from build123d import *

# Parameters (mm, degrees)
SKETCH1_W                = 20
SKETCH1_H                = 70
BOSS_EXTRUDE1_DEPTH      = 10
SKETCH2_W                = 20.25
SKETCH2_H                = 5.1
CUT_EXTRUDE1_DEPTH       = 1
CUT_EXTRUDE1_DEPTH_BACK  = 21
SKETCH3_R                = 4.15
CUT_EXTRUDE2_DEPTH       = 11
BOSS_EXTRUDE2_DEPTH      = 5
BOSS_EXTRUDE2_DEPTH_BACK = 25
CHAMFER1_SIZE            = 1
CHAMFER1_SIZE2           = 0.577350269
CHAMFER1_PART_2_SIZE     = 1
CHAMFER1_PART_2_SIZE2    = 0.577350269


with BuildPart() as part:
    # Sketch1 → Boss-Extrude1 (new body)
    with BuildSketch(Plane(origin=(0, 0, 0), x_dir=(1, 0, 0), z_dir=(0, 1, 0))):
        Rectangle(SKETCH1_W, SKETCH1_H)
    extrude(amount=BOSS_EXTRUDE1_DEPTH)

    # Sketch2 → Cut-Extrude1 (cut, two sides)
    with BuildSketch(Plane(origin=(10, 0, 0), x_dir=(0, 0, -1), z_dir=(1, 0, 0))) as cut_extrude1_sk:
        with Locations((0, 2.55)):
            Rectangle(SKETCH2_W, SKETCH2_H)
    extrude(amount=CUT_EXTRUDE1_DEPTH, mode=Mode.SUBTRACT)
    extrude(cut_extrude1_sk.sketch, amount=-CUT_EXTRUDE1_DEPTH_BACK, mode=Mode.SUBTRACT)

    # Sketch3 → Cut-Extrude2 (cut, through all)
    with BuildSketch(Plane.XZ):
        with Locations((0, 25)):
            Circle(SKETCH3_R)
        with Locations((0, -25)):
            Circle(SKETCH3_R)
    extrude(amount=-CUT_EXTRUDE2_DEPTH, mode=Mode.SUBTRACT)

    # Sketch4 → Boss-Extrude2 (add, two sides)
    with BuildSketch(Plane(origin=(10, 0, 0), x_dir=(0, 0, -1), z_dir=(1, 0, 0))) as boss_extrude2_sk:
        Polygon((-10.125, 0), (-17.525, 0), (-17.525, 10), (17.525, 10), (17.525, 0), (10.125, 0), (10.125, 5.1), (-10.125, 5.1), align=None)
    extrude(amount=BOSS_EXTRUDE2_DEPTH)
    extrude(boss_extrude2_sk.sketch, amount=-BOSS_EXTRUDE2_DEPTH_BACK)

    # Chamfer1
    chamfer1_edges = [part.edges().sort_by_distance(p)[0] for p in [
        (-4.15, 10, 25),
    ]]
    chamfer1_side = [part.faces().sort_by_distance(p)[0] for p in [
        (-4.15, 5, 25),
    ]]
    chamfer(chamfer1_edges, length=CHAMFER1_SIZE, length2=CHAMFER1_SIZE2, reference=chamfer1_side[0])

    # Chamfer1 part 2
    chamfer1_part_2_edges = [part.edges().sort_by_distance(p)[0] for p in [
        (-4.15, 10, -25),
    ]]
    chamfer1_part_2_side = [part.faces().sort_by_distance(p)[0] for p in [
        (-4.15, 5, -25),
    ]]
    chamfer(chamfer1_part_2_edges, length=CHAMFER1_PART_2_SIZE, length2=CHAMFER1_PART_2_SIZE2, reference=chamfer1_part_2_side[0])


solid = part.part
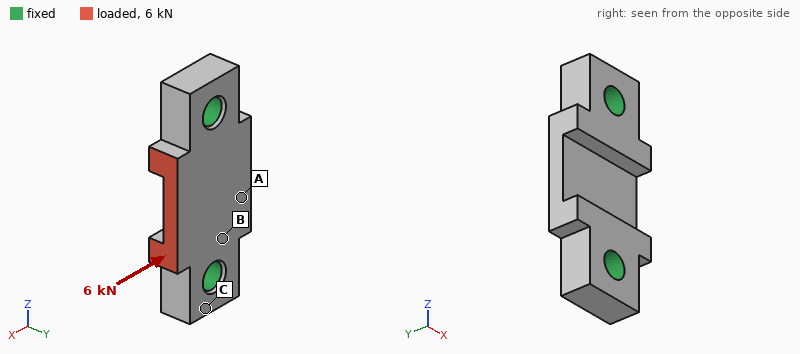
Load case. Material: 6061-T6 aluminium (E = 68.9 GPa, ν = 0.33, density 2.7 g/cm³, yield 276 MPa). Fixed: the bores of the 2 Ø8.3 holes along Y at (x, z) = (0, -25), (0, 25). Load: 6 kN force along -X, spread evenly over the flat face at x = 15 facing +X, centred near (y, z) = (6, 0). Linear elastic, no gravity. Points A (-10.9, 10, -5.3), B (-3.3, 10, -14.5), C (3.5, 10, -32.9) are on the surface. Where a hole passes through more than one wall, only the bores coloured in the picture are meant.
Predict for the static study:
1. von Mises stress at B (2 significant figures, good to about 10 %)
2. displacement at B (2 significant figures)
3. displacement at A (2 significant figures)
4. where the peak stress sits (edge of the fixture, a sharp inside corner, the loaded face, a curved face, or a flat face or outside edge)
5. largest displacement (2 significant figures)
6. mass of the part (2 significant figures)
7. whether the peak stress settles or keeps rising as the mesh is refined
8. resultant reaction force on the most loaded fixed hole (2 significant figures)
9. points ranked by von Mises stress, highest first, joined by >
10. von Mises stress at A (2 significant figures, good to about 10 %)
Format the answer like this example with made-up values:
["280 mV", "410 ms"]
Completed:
["31 MPa", "8.1 µm", "14 µm", "edge of the fixture", "21 µm", "36 g", "keeps rising", "3.0 kN", "B > A > C", "17 MPa"]
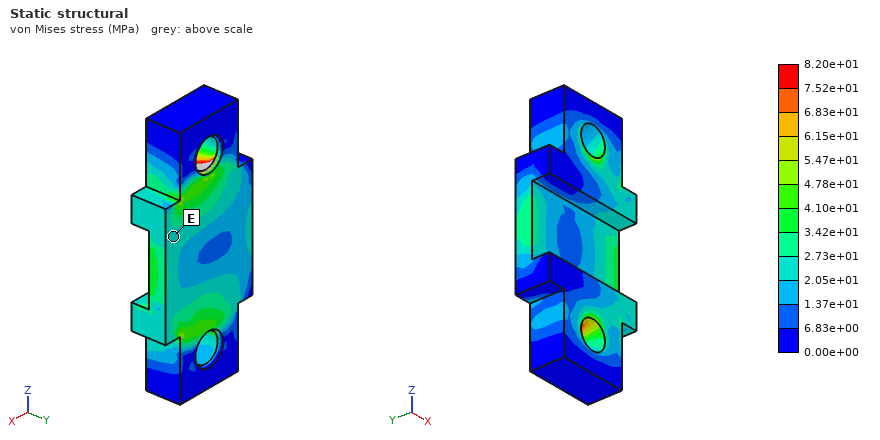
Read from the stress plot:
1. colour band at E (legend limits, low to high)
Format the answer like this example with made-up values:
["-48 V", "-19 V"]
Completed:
["2.05e+01 to 2.73e+01 MPa"]
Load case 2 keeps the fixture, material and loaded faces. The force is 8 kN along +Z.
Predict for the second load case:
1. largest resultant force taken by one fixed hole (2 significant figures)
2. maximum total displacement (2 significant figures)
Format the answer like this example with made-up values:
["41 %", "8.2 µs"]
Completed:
["4.6 kN", "32 µm"]
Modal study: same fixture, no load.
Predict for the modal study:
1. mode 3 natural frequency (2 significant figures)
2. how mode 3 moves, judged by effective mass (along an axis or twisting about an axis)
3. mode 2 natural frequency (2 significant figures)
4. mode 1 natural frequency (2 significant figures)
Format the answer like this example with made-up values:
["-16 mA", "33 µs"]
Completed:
["27 kHz", "along X", "18 kHz", "18 kHz"]
